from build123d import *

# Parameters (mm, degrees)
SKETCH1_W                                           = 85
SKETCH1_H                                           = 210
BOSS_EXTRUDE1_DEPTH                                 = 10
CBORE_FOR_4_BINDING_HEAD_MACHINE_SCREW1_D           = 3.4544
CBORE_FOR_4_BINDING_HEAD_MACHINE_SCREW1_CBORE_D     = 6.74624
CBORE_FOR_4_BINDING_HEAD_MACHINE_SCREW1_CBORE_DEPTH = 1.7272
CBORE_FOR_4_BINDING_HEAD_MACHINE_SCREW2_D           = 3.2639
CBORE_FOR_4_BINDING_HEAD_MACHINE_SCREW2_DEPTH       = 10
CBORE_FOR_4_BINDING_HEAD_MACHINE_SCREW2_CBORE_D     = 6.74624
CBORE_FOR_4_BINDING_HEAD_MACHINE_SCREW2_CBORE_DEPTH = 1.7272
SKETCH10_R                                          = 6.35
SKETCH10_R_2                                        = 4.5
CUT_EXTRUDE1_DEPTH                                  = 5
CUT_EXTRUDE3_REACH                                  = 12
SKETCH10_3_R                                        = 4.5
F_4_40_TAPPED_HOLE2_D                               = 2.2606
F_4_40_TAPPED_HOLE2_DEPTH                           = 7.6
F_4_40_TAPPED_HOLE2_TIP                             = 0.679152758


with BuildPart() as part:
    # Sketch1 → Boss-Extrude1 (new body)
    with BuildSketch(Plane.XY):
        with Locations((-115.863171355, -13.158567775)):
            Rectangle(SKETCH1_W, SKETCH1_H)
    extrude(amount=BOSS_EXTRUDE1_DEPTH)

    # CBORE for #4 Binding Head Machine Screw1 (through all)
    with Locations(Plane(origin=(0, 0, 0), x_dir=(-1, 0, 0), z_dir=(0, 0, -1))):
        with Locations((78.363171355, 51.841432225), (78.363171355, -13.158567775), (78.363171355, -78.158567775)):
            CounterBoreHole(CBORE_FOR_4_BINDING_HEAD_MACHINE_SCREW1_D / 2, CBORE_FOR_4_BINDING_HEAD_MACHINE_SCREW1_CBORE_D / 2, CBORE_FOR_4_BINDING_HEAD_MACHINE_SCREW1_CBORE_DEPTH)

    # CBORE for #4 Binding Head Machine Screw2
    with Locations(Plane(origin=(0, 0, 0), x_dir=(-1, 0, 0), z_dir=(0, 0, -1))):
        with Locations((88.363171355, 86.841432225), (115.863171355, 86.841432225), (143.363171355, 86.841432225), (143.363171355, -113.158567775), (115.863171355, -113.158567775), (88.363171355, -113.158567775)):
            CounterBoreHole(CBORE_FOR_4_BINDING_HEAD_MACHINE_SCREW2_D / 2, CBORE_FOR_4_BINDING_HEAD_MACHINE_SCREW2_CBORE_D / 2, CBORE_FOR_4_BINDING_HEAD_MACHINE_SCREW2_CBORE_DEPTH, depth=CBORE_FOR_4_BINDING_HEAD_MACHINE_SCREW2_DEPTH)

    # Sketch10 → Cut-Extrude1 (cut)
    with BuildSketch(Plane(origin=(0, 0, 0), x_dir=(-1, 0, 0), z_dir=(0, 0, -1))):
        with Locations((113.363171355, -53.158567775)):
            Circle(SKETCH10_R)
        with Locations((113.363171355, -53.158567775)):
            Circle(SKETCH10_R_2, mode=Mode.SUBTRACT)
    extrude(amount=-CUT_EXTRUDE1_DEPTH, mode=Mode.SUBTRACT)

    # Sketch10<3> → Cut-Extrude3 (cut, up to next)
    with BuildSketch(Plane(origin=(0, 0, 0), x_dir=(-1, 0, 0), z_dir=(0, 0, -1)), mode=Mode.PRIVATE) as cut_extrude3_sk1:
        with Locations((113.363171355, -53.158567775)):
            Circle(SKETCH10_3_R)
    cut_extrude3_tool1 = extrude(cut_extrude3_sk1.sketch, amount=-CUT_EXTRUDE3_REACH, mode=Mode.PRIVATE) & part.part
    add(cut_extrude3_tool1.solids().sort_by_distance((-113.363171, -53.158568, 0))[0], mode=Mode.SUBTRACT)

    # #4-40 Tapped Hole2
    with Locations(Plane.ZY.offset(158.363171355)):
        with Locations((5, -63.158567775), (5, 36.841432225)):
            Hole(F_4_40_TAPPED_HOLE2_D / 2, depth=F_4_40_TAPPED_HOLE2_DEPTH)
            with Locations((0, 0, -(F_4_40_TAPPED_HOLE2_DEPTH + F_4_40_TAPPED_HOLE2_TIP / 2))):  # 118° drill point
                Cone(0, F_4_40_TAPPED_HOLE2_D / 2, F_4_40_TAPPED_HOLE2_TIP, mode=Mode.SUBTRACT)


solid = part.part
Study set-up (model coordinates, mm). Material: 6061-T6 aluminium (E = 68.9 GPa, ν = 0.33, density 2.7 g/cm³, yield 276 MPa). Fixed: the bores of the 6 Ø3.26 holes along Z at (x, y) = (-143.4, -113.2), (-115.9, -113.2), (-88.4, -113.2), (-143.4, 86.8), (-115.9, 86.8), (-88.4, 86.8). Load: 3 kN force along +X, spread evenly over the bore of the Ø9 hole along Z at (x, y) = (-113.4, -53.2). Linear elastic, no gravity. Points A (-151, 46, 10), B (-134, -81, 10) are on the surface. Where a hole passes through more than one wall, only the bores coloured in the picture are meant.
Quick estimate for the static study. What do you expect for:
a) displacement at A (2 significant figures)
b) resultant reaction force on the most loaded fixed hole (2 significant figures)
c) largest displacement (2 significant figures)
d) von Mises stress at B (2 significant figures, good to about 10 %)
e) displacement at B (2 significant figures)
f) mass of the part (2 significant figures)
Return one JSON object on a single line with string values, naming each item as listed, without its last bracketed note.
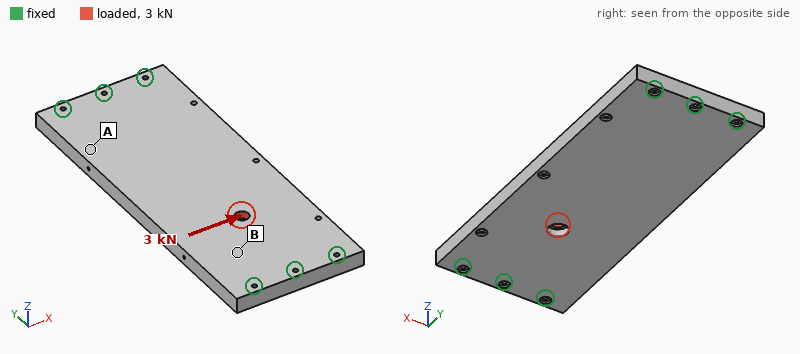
{"displacement at A": "6.2 µm", "resultant reaction force on the most loaded fixed hole": "1.2 kN", "largest displacement": "18 µm", "von Mises stress at B": "7.8 MPa", "displacement at B": "7.8 µm", "mass of the part": "480 g"}
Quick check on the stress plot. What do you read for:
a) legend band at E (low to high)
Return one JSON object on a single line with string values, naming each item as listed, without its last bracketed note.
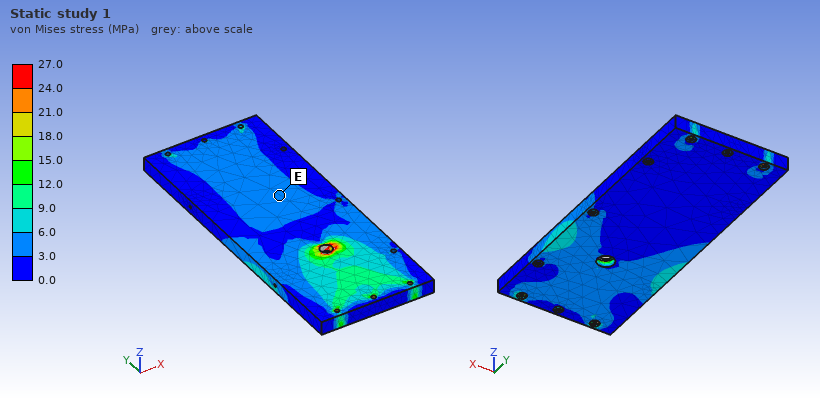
{"legend band at E": "3.0 to 6.0 MPa"}
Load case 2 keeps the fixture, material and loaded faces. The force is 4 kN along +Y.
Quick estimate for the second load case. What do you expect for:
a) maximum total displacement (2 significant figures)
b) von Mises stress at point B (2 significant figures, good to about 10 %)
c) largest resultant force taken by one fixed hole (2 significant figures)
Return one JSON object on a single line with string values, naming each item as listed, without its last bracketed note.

{"maximum total displacement": "14 µm", "von Mises stress at point B": "5.3 MPa", "largest resultant force taken by one fixed hole": "950 N"}
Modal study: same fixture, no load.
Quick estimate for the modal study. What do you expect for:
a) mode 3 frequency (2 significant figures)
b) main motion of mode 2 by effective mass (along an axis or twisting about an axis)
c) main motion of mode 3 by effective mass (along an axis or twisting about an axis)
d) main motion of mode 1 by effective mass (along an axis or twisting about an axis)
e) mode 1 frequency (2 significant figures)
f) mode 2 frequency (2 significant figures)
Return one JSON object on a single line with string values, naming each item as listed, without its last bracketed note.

{"mode 3 frequency": "3000 Hz", "main motion of mode 2 by effective mass": "twisting about Y", "main motion of mode 3 by effective mass": "twisting about X", "main motion of mode 1 by effective mass": "along Z", "mode 1 frequency": "1100 Hz", "mode 2 frequency": "2000 Hz"}
